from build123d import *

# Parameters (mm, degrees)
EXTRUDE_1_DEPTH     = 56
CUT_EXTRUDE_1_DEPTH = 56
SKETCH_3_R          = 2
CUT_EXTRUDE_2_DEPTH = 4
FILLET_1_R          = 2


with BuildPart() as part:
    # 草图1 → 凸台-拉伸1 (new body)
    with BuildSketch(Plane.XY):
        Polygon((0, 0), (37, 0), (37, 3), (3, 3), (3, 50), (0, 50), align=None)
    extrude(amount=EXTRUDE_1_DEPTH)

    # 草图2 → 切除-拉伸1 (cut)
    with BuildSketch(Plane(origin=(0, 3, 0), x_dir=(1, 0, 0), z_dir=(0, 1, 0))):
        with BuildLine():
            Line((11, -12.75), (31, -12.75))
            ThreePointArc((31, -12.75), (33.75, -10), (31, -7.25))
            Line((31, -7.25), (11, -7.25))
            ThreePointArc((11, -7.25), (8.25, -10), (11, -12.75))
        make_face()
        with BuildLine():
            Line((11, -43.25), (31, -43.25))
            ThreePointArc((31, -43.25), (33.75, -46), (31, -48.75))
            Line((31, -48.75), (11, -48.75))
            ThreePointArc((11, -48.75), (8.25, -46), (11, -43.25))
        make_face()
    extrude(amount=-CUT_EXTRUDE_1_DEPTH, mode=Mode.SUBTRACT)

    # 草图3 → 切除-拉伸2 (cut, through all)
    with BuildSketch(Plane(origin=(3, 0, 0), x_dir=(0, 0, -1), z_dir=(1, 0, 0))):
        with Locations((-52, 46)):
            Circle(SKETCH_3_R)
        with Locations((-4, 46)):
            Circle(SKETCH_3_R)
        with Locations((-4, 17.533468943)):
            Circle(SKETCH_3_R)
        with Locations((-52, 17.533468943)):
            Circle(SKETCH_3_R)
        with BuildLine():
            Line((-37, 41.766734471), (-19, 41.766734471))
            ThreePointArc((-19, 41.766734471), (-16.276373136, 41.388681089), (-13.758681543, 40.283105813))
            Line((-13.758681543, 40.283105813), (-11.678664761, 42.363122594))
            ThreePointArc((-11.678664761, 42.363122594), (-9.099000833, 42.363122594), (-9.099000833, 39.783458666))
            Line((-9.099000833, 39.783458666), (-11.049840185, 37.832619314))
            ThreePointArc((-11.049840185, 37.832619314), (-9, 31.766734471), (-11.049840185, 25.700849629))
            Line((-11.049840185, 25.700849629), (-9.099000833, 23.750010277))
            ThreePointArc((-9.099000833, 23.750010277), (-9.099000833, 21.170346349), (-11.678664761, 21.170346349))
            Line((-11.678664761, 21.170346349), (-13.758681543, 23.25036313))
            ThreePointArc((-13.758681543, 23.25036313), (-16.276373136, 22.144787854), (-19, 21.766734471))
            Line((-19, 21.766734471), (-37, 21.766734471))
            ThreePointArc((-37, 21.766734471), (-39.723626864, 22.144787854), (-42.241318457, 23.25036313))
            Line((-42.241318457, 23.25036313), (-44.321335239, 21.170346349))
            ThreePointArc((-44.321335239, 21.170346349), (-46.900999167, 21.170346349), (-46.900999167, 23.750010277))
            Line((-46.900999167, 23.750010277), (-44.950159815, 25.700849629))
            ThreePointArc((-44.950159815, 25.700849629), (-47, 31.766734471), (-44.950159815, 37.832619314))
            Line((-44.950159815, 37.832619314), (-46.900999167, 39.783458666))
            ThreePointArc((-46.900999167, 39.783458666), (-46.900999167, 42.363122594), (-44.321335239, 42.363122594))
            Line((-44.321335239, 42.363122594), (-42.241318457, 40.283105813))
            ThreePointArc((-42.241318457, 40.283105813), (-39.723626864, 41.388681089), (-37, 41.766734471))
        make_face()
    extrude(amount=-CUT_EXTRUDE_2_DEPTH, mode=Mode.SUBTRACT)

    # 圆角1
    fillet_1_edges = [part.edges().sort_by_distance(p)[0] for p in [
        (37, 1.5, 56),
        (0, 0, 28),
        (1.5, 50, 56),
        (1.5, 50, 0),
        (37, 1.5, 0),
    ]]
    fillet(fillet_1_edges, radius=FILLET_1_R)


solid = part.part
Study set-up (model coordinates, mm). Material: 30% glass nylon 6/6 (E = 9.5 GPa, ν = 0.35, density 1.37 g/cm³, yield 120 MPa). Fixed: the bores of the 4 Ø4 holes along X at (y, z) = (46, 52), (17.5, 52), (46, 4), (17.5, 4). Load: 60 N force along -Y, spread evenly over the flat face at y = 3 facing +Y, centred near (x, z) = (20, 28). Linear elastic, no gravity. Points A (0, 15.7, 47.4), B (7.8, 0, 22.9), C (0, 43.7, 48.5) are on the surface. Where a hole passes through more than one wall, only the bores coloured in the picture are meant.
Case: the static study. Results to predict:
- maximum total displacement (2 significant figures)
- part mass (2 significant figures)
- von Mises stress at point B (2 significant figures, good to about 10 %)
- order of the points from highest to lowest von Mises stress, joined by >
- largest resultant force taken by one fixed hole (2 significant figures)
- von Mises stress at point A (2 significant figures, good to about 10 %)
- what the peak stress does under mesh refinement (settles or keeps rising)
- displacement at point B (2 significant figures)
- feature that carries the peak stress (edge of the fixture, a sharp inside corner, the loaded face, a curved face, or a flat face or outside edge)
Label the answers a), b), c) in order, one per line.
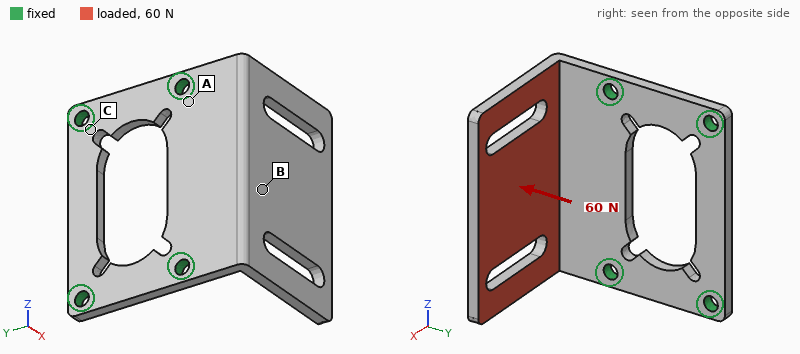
a) 0.95 mm
b) 15 g
c) 8.7 MPa
d) A > B > C
e) 32 N
f) 15 MPa
g) keeps rising
h) 0.24 mm
i) edge of the fixture
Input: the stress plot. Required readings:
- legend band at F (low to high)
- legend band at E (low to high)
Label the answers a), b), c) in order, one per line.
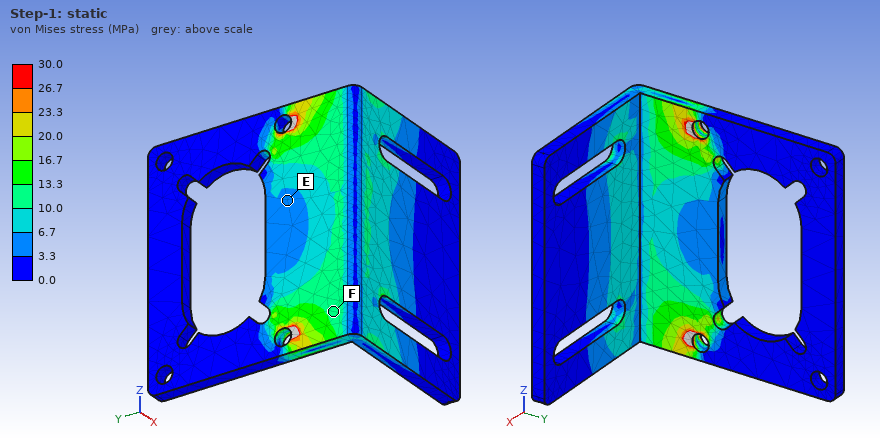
a) 10.0 to 13.3 MPa
b) 3.3 to 6.7 MPa
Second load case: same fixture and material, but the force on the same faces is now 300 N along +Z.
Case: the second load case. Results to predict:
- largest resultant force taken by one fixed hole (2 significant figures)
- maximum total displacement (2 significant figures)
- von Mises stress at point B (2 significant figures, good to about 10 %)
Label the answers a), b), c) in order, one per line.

a) 210 N
b) 0.67 mm
c) 10 MPa
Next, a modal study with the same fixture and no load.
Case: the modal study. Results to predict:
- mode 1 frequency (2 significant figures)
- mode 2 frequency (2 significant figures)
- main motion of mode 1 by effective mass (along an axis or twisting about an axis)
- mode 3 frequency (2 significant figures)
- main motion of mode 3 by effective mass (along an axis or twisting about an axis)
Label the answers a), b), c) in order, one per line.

a) 570 Hz
b) 1300 Hz
c) along Y
d) 1900 Hz
e) along X
